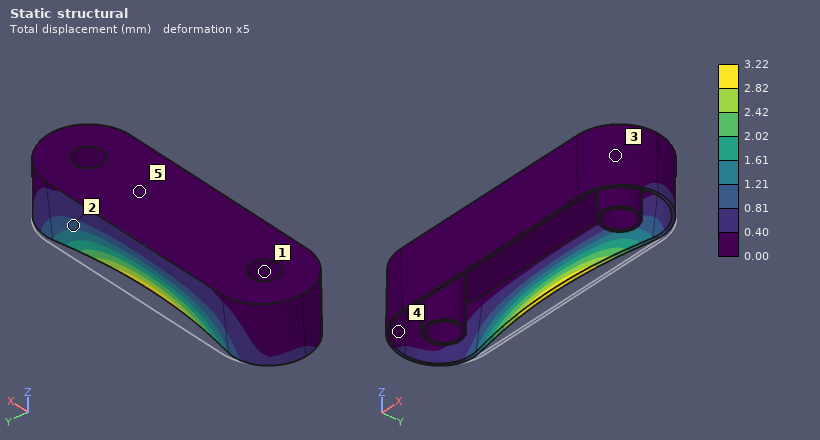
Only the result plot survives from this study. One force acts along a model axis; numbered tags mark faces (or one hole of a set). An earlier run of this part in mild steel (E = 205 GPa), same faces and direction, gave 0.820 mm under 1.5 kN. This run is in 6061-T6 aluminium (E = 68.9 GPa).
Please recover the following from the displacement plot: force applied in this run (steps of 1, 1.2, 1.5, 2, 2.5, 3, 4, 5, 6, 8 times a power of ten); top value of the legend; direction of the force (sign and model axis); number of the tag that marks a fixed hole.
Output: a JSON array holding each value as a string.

["2 kN", "3.22 mm", "-Y", "1"]
